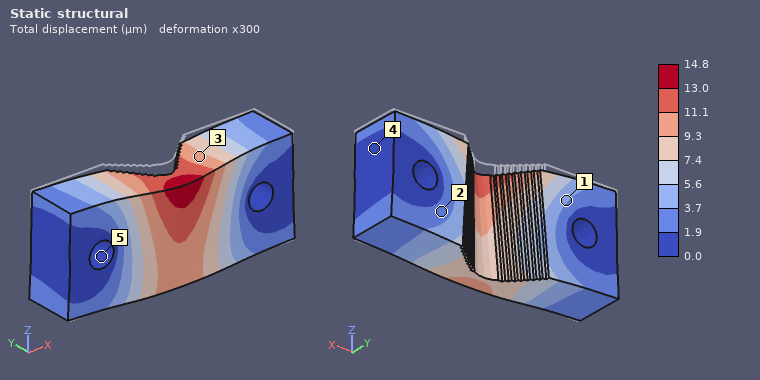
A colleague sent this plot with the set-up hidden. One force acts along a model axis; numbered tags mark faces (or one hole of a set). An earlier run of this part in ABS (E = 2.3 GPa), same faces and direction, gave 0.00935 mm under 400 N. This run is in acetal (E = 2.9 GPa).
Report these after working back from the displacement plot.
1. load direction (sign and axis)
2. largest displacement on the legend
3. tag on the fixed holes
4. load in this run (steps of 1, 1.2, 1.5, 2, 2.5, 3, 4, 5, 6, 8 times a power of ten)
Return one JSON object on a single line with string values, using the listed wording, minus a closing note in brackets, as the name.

{"load direction": "-Z", "largest displacement on the legend": "14.8 µm", "tag on the fixed holes": "5", "load in this run": "800 N"}
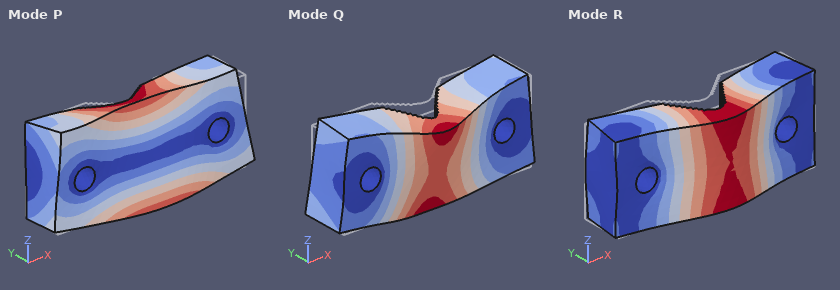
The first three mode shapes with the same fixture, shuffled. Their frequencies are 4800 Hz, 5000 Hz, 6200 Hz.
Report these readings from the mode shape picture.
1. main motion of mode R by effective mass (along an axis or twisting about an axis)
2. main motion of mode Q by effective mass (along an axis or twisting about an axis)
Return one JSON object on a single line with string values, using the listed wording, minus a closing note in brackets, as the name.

{"main motion of mode R by effective mass": "along Y", "main motion of mode Q by effective mass": "along Z"}
